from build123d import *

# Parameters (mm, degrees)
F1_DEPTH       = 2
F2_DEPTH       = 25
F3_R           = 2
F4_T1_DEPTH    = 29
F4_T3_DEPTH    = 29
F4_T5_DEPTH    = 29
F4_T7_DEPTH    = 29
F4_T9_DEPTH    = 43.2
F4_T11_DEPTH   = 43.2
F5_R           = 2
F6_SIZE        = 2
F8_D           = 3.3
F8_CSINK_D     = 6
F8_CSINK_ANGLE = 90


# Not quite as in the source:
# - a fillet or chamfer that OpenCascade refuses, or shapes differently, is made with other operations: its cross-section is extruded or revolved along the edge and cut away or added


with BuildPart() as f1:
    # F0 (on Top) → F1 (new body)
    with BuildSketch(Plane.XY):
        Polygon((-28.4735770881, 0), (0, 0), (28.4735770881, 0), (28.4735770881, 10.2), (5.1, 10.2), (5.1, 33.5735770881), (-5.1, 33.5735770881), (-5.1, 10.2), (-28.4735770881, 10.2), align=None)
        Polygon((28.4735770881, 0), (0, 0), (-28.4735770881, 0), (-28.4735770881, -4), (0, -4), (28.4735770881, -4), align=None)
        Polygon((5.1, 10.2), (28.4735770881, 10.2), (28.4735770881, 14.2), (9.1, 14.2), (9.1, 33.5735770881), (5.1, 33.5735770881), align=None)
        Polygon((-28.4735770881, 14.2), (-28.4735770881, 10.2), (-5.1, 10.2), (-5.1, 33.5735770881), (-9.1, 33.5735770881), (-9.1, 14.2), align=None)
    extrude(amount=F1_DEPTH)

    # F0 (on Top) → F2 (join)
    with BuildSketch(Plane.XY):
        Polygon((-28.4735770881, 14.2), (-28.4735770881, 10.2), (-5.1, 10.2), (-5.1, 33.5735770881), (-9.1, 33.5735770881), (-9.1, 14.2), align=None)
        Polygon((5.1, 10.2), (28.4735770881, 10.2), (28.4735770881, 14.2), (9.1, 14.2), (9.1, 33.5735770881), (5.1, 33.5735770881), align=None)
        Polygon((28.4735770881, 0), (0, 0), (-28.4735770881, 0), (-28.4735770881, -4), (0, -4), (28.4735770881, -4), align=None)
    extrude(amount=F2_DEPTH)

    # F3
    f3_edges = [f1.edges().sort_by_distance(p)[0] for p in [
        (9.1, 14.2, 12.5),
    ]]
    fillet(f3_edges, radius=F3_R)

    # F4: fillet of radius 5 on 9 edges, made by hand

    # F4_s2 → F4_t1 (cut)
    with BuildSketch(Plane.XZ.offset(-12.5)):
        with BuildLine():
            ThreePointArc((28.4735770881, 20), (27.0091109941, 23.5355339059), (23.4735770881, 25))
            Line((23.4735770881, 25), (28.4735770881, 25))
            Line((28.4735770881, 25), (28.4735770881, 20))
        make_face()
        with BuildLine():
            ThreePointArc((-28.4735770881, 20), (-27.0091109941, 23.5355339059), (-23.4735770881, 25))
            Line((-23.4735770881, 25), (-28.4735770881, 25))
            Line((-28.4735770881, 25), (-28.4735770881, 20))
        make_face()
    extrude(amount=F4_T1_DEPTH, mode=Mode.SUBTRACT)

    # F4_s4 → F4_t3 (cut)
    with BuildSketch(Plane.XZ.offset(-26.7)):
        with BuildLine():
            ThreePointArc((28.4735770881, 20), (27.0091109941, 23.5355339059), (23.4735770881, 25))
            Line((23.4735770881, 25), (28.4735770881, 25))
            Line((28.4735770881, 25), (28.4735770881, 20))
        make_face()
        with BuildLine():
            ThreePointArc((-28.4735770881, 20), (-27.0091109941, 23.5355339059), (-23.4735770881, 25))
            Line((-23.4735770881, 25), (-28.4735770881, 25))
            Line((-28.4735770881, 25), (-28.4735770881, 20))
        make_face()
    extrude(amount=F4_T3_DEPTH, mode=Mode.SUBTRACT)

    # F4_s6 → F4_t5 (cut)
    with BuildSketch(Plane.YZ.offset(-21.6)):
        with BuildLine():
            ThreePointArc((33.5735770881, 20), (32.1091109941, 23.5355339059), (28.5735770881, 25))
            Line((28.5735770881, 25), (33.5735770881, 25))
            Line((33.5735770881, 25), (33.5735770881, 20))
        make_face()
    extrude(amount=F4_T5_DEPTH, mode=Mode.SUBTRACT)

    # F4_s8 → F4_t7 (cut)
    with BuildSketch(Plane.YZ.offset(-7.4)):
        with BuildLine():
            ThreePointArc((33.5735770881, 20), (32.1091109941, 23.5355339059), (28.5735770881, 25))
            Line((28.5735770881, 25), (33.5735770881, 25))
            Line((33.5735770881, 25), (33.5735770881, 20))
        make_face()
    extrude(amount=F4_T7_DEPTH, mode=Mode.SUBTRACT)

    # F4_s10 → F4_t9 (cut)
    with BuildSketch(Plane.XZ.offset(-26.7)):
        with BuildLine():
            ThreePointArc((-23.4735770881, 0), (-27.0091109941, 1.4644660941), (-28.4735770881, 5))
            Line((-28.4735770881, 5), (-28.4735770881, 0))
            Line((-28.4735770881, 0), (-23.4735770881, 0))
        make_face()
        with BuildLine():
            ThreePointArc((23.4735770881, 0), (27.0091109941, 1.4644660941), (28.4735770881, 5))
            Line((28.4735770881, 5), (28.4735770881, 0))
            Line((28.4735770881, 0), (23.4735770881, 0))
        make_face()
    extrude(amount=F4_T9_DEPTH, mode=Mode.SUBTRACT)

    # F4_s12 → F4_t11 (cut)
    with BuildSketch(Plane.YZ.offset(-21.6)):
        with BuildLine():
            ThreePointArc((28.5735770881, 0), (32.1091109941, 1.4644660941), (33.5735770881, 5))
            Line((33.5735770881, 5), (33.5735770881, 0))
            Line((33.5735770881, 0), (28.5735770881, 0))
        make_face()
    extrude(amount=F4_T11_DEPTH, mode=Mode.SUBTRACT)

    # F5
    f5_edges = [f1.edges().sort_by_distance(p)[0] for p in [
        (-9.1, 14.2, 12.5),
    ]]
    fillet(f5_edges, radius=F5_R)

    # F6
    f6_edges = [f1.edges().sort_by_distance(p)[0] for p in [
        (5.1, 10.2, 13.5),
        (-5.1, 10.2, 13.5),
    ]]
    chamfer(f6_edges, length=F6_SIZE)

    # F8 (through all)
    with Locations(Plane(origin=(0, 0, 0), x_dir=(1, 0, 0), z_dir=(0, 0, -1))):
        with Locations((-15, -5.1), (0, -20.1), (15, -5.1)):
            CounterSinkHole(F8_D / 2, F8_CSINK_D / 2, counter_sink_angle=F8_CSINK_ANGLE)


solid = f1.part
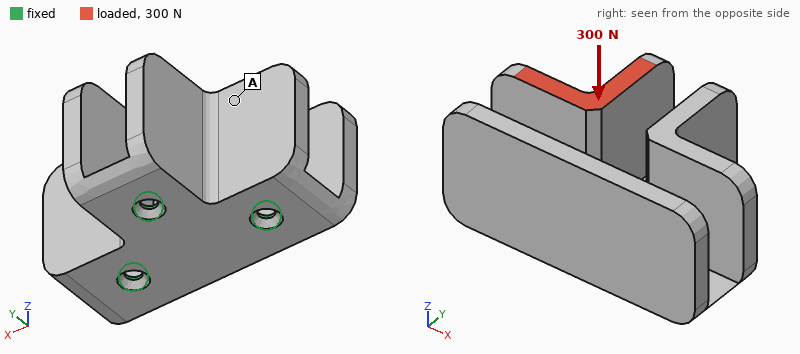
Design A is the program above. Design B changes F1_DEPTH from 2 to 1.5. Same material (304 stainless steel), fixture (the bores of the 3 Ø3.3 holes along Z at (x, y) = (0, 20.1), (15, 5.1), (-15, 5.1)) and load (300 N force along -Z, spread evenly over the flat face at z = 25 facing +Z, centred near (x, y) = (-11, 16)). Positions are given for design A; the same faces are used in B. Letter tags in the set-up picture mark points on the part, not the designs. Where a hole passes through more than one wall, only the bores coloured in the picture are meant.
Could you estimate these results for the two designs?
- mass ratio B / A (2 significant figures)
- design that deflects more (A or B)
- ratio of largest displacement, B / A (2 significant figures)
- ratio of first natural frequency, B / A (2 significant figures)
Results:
0.98
B
2.3
0.64
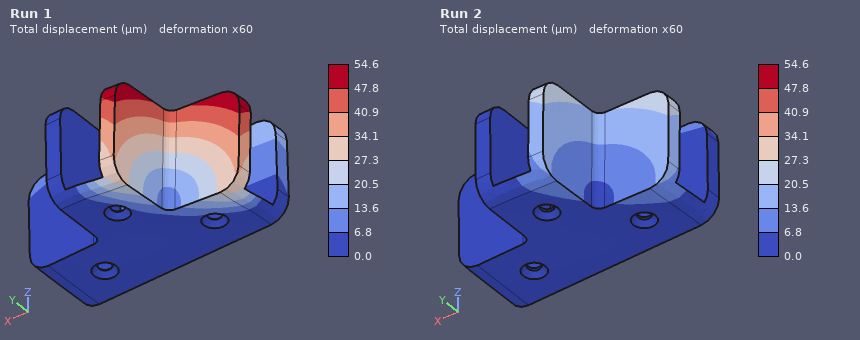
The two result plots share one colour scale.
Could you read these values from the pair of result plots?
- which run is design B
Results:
Run 1
